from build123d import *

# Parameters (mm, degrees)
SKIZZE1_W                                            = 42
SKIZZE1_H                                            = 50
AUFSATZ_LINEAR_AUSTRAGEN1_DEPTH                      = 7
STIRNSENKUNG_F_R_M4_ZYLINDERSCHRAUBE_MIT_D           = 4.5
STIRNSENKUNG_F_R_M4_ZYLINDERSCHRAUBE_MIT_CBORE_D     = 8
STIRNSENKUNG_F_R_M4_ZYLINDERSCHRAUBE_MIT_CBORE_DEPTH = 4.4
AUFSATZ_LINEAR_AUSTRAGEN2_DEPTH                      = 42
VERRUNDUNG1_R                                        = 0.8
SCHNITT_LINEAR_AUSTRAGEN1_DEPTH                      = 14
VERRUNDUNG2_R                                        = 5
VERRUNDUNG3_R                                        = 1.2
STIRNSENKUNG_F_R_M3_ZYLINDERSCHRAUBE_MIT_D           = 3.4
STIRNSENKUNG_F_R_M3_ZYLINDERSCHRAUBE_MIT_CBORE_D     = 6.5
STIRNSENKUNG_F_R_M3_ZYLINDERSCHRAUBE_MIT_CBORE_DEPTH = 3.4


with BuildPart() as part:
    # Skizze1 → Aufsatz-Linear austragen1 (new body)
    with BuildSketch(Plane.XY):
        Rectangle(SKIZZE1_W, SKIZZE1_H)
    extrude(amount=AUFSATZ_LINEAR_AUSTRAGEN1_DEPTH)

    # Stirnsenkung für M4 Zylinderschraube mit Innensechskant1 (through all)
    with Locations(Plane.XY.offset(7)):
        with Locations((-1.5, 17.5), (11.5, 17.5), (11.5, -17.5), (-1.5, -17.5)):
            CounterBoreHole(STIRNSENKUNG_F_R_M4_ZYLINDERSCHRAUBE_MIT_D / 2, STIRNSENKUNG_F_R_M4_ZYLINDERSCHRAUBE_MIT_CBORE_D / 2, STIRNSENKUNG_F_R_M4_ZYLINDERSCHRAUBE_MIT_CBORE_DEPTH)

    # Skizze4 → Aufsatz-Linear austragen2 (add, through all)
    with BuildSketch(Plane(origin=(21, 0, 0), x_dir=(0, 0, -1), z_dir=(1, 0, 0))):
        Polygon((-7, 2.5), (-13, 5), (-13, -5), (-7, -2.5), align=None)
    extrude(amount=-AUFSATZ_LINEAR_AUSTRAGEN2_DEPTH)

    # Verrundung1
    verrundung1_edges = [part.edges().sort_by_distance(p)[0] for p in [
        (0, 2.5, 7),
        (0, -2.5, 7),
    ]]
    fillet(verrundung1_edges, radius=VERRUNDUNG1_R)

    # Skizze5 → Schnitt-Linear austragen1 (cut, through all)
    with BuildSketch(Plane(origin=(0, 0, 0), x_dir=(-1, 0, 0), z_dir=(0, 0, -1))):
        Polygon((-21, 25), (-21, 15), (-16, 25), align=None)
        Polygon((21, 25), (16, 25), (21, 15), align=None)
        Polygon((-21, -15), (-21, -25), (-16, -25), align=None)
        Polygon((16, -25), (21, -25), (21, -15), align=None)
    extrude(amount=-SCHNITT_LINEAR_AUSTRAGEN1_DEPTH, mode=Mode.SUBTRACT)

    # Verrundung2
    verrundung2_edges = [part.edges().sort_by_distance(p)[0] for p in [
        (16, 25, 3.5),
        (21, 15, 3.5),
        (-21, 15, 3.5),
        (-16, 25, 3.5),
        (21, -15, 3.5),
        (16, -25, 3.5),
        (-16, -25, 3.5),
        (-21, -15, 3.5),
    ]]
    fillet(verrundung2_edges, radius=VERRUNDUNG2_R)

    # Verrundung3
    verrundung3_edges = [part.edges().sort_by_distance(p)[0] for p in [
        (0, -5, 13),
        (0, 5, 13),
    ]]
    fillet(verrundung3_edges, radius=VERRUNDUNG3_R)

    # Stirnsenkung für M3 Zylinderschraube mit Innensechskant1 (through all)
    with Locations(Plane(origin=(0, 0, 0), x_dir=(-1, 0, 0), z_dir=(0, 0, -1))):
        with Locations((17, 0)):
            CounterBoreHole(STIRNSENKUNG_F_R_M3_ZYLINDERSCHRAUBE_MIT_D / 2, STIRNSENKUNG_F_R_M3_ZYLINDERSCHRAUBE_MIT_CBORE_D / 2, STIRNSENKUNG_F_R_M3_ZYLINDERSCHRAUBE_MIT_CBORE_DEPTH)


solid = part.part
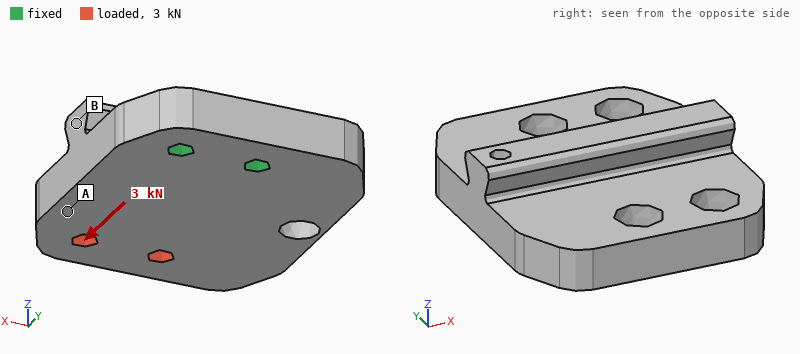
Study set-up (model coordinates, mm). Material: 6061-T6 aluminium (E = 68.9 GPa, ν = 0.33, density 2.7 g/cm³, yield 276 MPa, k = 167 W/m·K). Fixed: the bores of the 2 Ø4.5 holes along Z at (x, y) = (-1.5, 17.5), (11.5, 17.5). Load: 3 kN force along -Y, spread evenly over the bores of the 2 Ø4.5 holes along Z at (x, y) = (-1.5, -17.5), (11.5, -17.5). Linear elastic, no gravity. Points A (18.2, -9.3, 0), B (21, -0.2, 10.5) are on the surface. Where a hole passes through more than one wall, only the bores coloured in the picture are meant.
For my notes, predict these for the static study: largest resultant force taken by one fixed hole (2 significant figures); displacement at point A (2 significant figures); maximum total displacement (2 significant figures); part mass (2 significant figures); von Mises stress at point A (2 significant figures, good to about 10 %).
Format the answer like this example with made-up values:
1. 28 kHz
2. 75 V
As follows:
1. 1.5 kN
2. 24 µm
3. 64 µm
4. 39 g
5. 33 MPa
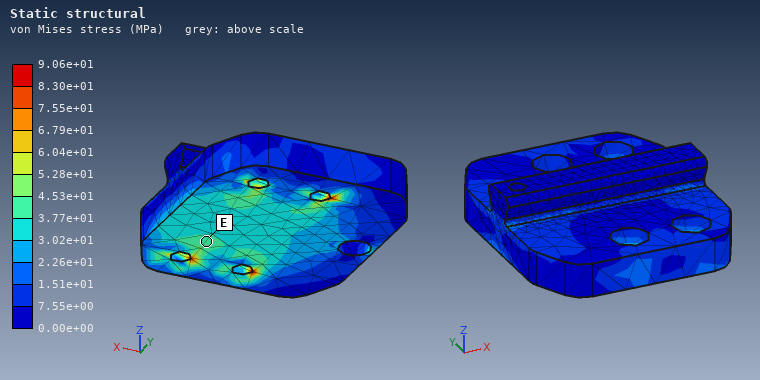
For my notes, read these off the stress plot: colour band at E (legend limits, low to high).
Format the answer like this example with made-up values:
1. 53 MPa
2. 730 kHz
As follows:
1. 3.77e+01 to 4.53e+01 MPa
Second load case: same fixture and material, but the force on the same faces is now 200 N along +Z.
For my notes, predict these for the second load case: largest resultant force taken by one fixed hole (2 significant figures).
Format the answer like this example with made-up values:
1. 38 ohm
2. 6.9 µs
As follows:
1. 130 N
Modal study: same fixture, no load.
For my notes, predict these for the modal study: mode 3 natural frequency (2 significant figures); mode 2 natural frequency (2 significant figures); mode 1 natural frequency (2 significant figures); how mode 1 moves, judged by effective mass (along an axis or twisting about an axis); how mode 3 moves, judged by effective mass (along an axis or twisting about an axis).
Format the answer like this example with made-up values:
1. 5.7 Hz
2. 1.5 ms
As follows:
1. 6000 Hz
2. 5300 Hz
3. 1900 Hz
4. along Z
5. along X
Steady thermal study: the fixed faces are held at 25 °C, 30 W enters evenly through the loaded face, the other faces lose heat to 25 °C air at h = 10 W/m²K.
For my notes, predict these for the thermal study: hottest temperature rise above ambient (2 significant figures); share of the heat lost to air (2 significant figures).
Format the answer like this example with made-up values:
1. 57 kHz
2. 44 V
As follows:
1. 35 K
2. 3.3 %
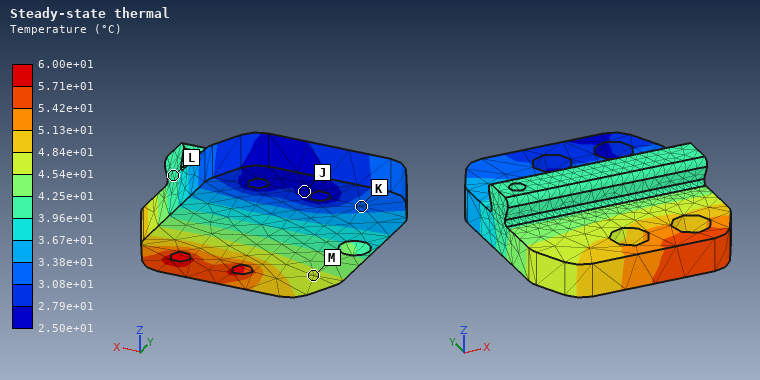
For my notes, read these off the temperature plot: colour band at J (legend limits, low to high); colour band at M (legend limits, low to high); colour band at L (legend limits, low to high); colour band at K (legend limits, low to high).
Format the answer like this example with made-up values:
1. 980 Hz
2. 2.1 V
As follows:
1. 2.50e+01 to 2.79e+01 °C
2. 4.54e+01 to 4.84e+01 °C
3. 3.96e+01 to 4.25e+01 °C
4. 3.08e+01 to 3.38e+01 °C
